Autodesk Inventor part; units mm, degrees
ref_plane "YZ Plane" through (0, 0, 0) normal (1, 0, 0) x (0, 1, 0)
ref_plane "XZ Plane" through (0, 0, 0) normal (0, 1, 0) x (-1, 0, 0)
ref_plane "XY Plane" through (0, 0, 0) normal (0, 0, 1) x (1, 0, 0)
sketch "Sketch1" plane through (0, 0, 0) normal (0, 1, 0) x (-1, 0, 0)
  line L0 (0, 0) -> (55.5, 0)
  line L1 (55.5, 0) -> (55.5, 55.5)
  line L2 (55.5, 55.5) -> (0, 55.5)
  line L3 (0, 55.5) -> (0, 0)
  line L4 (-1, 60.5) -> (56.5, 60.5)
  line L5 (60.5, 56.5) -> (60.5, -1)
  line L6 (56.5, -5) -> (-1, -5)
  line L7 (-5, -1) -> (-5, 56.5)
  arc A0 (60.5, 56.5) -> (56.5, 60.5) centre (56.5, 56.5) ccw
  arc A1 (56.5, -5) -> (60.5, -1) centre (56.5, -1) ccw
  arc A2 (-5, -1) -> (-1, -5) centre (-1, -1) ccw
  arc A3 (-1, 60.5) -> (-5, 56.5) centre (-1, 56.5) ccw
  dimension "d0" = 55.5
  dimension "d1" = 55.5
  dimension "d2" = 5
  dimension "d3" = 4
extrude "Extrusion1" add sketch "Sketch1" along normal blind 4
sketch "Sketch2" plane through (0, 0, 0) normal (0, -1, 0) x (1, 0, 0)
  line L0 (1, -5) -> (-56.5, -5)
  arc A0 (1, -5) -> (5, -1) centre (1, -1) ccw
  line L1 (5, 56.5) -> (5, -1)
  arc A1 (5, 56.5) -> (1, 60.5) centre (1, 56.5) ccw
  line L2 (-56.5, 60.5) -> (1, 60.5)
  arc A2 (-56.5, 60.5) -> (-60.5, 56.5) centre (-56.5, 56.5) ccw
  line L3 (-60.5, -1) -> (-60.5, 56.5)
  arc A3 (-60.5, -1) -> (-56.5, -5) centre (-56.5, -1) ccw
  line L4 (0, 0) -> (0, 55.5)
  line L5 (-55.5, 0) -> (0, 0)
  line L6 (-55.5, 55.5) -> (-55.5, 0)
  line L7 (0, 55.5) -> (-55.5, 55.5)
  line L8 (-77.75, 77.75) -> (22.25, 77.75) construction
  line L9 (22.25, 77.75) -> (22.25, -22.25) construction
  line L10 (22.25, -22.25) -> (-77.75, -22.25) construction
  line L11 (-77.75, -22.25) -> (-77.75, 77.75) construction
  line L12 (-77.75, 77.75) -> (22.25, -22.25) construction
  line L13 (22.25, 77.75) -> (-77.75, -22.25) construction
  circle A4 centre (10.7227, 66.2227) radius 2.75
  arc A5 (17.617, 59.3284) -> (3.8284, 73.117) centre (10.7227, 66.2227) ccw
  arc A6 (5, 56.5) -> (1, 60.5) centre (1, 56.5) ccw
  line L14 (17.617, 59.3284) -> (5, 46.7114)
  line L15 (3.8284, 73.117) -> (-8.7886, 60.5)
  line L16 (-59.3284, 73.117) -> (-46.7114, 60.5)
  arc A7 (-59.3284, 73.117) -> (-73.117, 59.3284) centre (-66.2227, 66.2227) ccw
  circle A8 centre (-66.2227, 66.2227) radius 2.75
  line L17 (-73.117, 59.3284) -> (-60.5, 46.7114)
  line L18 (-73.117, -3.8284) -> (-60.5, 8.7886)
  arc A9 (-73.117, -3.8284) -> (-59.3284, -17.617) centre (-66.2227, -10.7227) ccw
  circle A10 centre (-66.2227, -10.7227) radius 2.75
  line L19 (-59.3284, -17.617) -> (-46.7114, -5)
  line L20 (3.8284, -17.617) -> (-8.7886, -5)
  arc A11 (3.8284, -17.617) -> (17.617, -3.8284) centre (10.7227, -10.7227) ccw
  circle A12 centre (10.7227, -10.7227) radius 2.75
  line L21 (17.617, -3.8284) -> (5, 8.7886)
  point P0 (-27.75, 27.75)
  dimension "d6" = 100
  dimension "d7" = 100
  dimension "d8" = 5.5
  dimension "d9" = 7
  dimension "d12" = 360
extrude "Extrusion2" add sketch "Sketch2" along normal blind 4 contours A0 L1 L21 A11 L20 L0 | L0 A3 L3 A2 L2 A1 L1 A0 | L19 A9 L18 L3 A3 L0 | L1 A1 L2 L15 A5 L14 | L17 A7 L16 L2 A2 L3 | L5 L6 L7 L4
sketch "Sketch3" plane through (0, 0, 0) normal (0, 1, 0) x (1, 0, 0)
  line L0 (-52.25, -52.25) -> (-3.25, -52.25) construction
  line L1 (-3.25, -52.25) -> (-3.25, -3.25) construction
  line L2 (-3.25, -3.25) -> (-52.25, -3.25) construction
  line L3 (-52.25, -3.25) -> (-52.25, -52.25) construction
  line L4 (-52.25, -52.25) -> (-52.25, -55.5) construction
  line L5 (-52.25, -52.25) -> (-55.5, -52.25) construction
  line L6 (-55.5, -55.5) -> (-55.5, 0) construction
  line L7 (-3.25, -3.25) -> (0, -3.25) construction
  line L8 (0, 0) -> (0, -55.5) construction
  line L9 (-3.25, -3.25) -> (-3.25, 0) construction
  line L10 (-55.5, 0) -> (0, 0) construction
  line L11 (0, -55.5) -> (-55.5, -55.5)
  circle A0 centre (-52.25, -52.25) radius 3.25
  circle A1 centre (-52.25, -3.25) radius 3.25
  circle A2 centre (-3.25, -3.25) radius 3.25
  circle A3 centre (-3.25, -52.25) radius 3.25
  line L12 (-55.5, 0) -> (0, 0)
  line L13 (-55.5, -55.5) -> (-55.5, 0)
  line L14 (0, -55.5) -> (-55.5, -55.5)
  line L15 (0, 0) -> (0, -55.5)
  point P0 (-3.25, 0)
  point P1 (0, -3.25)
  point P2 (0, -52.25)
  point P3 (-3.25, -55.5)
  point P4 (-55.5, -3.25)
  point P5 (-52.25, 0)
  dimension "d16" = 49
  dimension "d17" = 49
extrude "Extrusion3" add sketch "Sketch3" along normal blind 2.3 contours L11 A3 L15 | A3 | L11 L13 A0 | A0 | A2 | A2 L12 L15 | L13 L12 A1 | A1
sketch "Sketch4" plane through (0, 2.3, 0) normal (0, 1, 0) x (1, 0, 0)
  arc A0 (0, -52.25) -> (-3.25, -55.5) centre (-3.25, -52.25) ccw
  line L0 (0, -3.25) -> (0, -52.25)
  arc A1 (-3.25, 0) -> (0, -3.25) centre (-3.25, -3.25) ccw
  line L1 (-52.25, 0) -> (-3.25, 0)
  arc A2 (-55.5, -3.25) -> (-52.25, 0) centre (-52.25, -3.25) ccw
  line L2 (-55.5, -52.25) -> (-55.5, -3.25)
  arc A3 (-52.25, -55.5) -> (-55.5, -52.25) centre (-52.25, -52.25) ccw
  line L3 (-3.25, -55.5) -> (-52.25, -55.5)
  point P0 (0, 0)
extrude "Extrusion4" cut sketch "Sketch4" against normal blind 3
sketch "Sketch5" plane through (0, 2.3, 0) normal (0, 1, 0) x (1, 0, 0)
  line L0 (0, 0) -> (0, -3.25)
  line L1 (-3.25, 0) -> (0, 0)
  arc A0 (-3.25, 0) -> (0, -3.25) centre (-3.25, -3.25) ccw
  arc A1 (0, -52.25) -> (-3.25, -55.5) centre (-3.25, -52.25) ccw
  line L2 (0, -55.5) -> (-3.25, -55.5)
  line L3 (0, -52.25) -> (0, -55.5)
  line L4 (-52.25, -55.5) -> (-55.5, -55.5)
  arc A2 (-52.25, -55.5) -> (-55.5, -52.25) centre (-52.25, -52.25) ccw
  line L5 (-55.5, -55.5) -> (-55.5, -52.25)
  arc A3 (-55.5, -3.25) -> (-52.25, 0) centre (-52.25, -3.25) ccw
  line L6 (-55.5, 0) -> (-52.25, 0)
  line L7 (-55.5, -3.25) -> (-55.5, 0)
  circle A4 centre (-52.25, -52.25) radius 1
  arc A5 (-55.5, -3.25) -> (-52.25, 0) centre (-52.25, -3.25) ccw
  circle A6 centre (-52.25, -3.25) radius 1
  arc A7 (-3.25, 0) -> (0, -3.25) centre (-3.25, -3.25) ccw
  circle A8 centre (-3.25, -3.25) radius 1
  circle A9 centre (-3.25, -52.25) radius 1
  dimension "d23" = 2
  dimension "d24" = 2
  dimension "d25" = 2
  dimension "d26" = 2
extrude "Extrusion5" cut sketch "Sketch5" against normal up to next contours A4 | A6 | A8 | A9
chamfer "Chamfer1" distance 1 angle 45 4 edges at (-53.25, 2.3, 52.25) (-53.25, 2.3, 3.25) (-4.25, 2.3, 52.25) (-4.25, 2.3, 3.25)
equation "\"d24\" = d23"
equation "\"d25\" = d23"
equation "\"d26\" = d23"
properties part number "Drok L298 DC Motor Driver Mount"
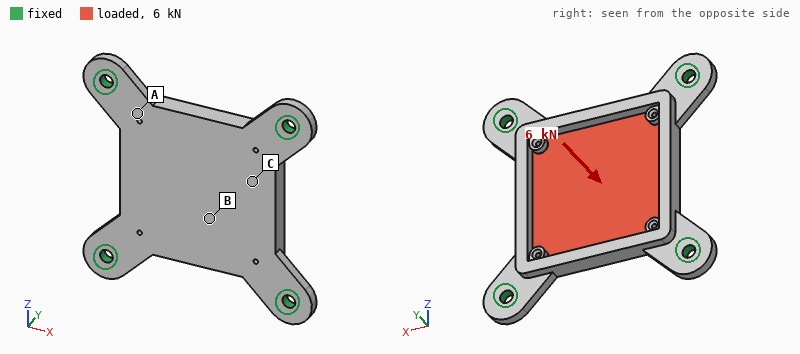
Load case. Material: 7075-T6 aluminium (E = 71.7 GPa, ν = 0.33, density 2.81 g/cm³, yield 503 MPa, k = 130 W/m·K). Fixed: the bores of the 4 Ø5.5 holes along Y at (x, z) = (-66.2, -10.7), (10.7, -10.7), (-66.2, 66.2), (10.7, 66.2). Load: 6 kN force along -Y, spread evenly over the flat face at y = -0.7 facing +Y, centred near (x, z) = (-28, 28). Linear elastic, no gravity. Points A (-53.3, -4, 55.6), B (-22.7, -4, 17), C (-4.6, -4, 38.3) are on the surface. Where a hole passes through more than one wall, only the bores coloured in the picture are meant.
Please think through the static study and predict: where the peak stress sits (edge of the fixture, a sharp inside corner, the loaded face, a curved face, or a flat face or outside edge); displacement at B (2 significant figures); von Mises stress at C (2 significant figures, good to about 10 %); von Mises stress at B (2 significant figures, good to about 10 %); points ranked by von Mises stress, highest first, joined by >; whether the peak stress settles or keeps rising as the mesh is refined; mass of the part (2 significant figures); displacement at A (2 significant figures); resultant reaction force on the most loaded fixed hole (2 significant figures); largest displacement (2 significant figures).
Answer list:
edge of the fixture
0.65 mm
100 MPa
180 MPa
B > C > A
keeps rising
74 g
0.20 mm
1.8 kN
0.72 mm
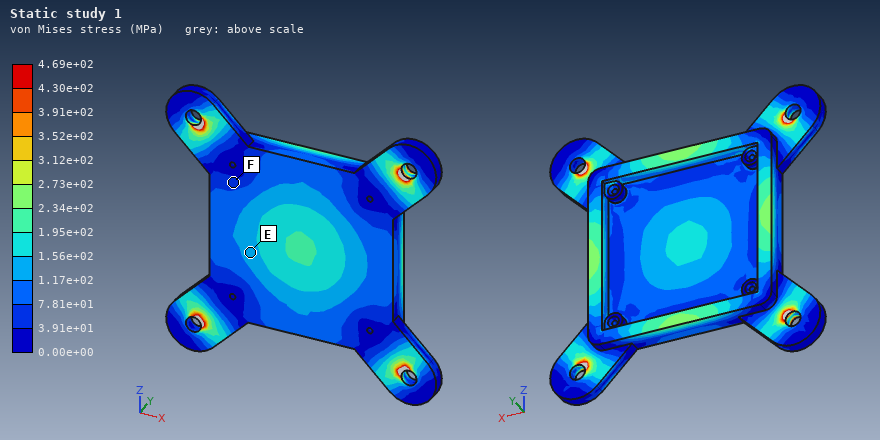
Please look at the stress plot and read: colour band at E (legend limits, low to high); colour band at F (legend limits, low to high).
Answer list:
1.17e+02 to 1.56e+02 MPa
3.91e+01 to 7.81e+01 MPa
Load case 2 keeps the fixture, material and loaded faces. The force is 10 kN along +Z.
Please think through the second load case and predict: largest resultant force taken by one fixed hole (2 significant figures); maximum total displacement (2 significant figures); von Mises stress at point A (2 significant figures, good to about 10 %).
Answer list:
3.0 kN
38 µm
35 MPa
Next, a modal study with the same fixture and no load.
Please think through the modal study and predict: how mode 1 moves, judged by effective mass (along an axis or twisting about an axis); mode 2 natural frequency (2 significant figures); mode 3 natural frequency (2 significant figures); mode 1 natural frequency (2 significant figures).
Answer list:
along Y
5200 Hz
5200 Hz
2800 Hz
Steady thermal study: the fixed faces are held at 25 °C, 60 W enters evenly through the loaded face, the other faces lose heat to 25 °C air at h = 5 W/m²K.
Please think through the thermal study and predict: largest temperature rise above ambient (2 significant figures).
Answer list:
42 K
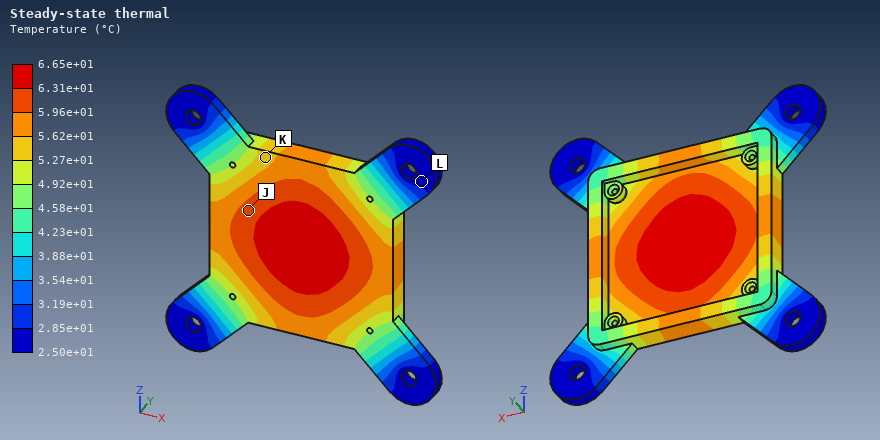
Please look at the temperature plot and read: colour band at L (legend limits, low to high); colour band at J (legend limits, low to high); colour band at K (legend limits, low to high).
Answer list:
2.50e+01 to 2.85e+01 °C
5.96e+01 to 6.31e+01 °C
5.27e+01 to 5.62e+01 °C
